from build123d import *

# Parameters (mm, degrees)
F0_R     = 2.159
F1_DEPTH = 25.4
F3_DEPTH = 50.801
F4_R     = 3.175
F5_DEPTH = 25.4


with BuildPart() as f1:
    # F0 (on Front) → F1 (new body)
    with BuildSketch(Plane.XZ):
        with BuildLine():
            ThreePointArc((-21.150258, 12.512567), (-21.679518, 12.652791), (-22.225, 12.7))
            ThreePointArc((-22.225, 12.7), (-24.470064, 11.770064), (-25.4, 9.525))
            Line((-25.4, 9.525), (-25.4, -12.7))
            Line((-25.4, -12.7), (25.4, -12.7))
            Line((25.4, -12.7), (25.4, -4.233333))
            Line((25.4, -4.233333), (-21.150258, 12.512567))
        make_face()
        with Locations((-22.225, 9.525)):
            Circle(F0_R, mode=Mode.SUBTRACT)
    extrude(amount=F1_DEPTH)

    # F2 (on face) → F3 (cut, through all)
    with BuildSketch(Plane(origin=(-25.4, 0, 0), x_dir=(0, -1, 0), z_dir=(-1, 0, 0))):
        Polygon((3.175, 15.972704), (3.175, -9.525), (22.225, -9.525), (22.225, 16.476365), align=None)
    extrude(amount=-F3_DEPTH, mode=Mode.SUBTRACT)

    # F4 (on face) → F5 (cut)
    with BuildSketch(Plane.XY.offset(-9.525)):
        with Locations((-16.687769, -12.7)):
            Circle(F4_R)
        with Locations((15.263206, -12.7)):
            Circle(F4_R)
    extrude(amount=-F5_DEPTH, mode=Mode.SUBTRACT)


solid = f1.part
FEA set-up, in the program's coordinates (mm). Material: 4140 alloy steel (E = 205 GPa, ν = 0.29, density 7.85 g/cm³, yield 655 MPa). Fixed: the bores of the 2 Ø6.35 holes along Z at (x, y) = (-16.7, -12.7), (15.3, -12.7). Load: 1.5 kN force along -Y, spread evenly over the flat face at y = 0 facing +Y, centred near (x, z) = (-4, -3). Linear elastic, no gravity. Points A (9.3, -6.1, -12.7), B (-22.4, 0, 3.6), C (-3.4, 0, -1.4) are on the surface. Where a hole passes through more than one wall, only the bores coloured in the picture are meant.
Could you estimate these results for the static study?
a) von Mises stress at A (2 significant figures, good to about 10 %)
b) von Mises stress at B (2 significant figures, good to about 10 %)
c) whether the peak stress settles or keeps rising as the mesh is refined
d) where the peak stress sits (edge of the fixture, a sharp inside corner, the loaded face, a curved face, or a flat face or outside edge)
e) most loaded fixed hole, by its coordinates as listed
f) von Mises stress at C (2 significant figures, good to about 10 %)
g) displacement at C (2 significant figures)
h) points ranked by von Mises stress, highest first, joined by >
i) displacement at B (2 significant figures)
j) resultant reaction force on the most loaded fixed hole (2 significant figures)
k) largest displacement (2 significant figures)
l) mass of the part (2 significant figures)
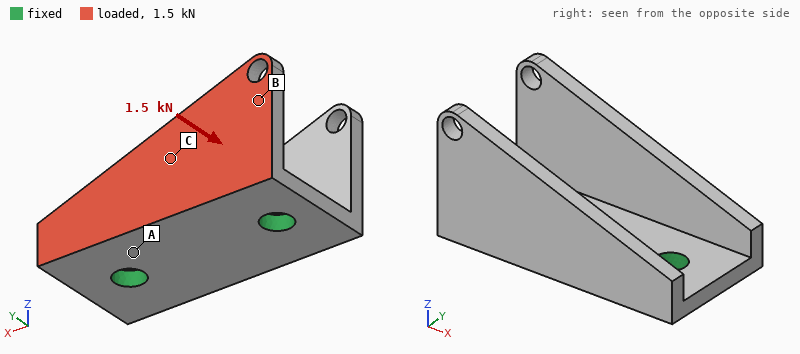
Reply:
96 MPa
23 MPa
keeps rising
edge of the fixture
(-16.7, -12.7)
56 MPa
0.060 mm
A > C > B
0.11 mm
900 N
0.18 mm
66 g
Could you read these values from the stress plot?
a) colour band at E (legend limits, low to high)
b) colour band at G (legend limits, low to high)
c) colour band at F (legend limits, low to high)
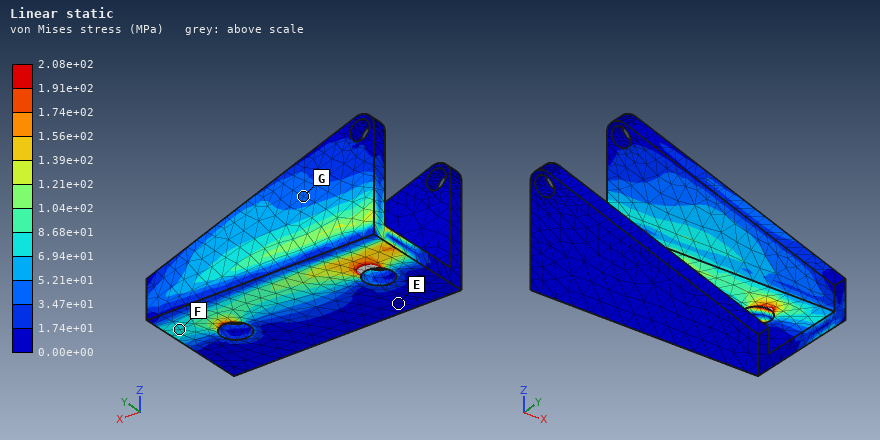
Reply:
0.00e+00 to 1.74e+01 MPa
3.47e+01 to 5.21e+01 MPa
6.94e+01 to 8.68e+01 MPa
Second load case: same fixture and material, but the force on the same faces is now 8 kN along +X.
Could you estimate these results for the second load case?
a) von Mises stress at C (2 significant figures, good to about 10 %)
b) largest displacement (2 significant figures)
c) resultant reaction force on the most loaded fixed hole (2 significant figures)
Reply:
52 MPa
80 µm
5.2 kN
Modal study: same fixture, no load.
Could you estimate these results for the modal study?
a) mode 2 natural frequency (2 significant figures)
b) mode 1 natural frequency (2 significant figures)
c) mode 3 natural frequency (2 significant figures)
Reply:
4300 Hz
4200 Hz
8700 Hz
